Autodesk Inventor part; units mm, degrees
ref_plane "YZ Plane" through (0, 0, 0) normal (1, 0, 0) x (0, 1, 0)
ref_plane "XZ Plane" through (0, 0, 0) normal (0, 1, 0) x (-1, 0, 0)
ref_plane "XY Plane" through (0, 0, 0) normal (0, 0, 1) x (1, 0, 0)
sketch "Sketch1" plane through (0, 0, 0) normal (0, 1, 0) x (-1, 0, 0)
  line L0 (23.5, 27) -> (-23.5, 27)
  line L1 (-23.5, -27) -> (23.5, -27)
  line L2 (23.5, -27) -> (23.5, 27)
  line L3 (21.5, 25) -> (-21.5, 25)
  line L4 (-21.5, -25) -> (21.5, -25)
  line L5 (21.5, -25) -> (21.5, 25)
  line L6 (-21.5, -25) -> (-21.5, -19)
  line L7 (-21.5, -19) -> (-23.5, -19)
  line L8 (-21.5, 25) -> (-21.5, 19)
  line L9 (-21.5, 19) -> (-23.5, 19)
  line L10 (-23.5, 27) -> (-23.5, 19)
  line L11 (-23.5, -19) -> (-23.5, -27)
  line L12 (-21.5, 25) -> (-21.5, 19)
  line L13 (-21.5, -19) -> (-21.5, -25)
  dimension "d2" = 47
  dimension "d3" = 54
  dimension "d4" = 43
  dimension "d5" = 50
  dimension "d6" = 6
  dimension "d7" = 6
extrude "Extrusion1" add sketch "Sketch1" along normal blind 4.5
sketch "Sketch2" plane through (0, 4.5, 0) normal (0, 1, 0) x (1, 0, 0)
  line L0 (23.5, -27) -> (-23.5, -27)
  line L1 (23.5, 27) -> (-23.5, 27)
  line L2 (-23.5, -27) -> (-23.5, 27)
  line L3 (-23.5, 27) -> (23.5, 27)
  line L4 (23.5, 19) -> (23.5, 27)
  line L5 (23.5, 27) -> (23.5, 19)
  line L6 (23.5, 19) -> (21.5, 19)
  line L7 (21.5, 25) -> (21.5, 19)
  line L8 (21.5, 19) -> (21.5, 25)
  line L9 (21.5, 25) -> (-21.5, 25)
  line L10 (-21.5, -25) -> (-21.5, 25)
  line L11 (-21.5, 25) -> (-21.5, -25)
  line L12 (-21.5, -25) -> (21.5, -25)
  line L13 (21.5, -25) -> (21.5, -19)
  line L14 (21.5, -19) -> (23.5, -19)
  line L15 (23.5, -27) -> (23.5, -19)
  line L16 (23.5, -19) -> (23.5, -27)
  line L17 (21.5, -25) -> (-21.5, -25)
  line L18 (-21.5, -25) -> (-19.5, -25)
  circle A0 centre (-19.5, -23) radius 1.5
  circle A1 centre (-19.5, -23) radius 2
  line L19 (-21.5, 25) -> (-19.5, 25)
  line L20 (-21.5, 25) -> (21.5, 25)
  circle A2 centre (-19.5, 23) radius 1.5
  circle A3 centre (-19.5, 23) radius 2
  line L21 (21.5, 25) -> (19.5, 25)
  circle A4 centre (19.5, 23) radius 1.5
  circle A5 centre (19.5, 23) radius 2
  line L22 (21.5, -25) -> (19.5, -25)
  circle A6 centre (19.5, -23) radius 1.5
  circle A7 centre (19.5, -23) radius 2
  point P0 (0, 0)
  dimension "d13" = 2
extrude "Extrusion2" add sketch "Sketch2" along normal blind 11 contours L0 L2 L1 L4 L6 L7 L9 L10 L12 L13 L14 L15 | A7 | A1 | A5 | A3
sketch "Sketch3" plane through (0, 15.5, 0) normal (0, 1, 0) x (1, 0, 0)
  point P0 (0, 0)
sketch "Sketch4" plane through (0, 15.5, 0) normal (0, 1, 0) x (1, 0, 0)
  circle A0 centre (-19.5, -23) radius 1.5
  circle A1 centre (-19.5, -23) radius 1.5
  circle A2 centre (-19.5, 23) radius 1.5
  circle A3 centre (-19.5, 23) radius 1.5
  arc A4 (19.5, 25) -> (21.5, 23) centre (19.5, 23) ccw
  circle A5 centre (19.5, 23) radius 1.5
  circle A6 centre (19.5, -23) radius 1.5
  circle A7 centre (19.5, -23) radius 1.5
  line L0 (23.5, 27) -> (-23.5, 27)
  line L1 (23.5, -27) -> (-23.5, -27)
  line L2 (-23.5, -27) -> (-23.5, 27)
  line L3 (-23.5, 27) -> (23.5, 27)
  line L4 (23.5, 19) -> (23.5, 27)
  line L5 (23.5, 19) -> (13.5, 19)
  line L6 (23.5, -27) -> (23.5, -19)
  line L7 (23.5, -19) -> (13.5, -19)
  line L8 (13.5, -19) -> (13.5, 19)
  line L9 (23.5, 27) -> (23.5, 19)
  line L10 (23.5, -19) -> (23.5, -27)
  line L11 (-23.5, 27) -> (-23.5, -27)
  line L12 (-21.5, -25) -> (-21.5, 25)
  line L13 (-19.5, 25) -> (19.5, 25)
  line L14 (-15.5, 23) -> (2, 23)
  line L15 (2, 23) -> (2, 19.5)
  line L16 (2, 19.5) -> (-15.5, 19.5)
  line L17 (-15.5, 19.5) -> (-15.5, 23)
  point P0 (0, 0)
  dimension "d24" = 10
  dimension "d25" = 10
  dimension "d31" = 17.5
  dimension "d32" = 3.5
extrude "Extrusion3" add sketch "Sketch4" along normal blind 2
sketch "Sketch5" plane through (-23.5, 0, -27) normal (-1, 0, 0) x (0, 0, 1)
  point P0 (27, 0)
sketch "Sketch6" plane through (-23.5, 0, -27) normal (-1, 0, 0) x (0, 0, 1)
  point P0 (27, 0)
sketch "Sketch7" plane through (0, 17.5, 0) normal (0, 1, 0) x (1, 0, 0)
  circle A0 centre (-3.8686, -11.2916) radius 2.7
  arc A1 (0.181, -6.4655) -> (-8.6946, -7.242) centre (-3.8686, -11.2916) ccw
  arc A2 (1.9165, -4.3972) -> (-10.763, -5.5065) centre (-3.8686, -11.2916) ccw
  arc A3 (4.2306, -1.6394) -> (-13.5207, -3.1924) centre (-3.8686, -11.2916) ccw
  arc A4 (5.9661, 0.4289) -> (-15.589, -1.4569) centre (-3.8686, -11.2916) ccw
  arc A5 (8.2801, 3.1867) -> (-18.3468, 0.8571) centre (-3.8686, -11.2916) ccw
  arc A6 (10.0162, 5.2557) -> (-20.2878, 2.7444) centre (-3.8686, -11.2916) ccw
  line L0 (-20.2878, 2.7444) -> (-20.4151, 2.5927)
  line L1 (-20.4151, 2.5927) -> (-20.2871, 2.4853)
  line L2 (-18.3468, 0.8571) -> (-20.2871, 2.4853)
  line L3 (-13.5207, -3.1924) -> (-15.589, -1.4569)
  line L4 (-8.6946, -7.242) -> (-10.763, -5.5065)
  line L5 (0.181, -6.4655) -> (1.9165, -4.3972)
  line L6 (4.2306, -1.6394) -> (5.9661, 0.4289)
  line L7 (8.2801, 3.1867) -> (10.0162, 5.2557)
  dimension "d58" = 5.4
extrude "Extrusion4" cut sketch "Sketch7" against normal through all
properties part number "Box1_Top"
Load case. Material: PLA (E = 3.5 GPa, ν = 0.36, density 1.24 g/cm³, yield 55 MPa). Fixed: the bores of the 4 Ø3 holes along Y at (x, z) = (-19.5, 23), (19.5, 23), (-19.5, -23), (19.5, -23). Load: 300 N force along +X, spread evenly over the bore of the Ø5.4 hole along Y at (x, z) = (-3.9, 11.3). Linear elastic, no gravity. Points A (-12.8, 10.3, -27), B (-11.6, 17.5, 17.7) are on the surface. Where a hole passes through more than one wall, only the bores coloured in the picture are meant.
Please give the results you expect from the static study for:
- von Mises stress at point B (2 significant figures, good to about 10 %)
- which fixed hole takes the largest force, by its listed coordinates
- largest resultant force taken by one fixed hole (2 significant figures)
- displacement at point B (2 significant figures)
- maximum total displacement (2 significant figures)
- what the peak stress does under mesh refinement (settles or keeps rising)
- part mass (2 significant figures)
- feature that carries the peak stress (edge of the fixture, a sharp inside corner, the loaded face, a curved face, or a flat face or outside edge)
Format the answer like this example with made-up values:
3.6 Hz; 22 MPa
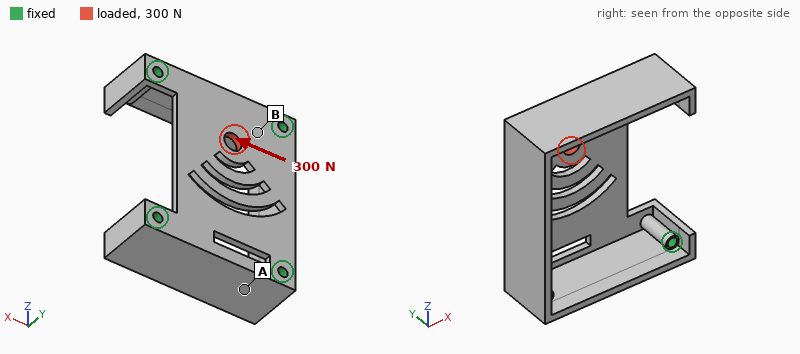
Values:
6.8 MPa; (-19.5, 23); 170 N; 26 µm; 70 µm; keeps rising; 11 g; edge of the fixture
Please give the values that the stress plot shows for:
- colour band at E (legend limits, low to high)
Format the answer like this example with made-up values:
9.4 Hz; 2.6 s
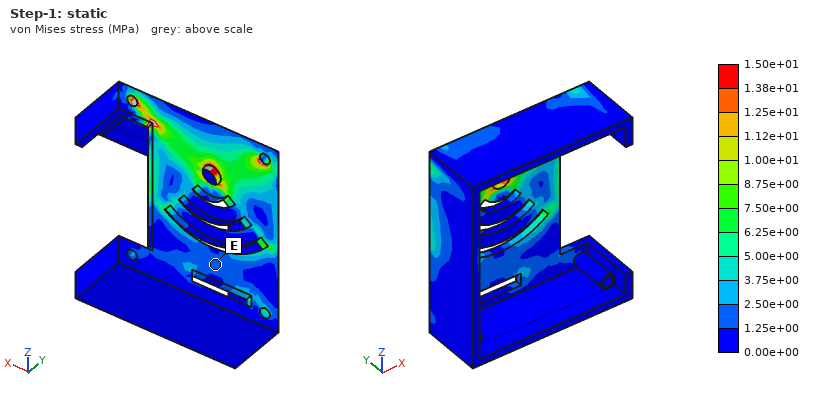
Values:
1.25e+00 to 2.50e+00 MPa
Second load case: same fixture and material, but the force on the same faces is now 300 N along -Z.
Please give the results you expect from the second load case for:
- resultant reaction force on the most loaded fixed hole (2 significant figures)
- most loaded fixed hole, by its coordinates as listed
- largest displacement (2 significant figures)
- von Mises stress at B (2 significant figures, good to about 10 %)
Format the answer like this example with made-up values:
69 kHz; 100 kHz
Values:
180 N; (-19.5, 23); 95 µm; 8.3 MPa
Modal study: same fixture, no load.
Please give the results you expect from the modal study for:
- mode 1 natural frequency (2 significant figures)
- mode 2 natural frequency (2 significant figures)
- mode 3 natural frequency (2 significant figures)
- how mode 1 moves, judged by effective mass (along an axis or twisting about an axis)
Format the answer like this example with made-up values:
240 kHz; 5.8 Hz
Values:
1300 Hz; 2200 Hz; 2500 Hz; along Y
